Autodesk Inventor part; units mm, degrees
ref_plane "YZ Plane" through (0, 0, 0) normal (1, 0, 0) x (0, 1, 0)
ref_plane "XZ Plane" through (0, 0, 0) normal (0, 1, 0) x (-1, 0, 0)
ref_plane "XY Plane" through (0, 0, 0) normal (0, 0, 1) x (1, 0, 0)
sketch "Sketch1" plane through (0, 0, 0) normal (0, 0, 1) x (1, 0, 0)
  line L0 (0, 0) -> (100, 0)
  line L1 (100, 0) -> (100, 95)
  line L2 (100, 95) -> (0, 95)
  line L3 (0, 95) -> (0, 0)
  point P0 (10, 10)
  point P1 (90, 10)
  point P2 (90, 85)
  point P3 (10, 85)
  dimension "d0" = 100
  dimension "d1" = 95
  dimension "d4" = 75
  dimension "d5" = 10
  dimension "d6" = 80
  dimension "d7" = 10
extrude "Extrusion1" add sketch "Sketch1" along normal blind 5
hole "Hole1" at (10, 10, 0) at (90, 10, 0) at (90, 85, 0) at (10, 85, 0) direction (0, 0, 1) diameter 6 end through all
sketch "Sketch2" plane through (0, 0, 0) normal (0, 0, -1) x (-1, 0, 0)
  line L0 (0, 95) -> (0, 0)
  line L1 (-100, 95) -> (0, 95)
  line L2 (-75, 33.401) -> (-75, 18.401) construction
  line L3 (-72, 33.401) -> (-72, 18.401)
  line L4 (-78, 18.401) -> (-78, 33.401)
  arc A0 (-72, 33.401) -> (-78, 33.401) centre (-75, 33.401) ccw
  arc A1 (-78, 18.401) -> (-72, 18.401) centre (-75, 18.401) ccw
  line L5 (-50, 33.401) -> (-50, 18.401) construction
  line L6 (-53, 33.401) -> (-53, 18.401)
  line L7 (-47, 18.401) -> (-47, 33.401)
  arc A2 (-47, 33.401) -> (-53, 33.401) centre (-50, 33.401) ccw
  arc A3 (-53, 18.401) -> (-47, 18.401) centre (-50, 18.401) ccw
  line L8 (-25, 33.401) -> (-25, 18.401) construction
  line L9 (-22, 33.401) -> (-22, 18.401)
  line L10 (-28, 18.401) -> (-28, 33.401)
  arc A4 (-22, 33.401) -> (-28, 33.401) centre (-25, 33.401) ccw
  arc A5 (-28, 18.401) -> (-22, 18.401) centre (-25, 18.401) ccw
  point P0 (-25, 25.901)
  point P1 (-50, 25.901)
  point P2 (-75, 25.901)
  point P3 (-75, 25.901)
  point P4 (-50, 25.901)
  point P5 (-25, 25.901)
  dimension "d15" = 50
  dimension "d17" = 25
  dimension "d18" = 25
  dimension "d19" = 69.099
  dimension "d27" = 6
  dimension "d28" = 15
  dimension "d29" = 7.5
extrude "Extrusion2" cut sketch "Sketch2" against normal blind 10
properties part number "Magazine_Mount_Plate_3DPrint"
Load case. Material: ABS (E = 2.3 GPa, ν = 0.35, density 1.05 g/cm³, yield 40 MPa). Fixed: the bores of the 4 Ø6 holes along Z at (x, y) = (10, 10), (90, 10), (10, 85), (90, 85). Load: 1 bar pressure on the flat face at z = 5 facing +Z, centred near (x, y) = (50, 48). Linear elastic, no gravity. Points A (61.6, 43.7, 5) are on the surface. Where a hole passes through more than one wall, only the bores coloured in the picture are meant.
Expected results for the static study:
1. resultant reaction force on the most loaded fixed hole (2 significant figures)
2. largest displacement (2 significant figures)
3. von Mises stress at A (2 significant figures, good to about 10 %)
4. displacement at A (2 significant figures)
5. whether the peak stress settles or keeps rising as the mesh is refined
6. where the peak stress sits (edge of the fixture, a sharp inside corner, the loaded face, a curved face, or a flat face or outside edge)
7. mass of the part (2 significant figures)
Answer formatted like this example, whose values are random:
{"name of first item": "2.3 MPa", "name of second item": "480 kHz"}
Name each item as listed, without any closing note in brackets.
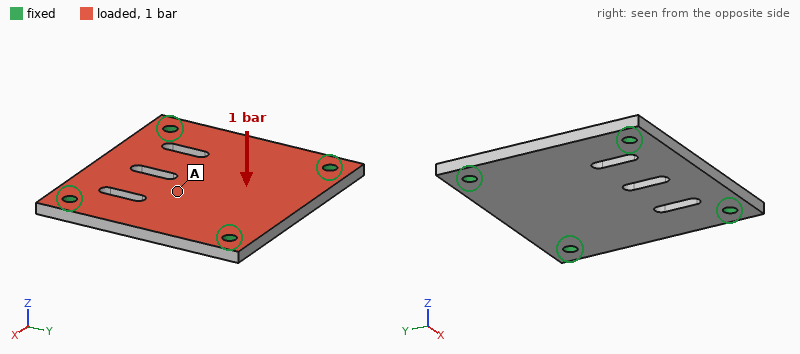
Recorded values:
{"resultant reaction force on the most loaded fixed hole": "230 N", "largest displacement": "1.0 mm", "von Mises stress at A": "6.6 MPa", "displacement at A": "0.92 mm", "whether the peak stress settles or keeps rising as the mesh is refined": "keeps rising", "where the peak stress sits": "edge of the fixture", "mass of the part": "47 g"}
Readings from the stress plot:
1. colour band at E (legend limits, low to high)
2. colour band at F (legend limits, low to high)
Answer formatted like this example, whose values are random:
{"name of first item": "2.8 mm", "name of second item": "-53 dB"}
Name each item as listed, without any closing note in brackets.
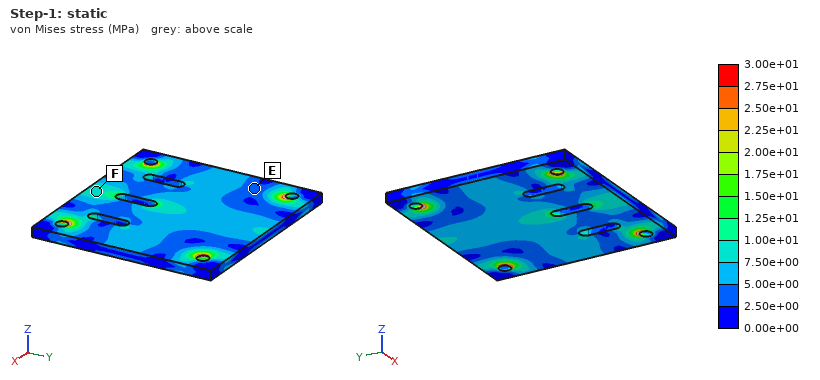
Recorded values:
{"colour band at E": "2.50e+00 to 5.00e+00 MPa", "colour band at F": "7.50e+00 to 1.00e+01 MPa"}
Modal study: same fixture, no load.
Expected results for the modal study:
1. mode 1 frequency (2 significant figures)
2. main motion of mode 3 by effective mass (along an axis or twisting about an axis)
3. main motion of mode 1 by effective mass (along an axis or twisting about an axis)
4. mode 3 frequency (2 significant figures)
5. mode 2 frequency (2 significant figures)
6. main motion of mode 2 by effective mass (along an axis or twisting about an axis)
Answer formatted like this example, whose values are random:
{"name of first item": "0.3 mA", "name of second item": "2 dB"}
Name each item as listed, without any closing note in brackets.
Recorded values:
{"mode 1 frequency": "850 Hz", "main motion of mode 3 by effective mass": "twisting about Y", "main motion of mode 1 by effective mass": "along Z", "mode 3 frequency": "1500 Hz", "mode 2 frequency": "1300 Hz", "main motion of mode 2 by effective mass": "twisting about X"}
